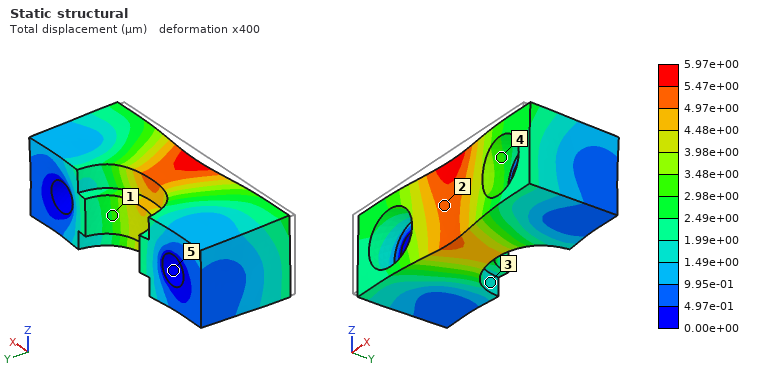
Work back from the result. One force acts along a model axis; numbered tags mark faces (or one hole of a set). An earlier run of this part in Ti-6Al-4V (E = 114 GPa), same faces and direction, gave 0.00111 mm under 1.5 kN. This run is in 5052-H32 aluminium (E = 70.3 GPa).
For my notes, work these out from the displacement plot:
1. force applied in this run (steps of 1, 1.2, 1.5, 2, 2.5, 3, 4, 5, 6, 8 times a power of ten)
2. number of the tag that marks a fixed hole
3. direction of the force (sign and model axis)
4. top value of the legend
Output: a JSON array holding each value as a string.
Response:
["5 kN", "5", "+Y", "5.97e+00 µm"]
